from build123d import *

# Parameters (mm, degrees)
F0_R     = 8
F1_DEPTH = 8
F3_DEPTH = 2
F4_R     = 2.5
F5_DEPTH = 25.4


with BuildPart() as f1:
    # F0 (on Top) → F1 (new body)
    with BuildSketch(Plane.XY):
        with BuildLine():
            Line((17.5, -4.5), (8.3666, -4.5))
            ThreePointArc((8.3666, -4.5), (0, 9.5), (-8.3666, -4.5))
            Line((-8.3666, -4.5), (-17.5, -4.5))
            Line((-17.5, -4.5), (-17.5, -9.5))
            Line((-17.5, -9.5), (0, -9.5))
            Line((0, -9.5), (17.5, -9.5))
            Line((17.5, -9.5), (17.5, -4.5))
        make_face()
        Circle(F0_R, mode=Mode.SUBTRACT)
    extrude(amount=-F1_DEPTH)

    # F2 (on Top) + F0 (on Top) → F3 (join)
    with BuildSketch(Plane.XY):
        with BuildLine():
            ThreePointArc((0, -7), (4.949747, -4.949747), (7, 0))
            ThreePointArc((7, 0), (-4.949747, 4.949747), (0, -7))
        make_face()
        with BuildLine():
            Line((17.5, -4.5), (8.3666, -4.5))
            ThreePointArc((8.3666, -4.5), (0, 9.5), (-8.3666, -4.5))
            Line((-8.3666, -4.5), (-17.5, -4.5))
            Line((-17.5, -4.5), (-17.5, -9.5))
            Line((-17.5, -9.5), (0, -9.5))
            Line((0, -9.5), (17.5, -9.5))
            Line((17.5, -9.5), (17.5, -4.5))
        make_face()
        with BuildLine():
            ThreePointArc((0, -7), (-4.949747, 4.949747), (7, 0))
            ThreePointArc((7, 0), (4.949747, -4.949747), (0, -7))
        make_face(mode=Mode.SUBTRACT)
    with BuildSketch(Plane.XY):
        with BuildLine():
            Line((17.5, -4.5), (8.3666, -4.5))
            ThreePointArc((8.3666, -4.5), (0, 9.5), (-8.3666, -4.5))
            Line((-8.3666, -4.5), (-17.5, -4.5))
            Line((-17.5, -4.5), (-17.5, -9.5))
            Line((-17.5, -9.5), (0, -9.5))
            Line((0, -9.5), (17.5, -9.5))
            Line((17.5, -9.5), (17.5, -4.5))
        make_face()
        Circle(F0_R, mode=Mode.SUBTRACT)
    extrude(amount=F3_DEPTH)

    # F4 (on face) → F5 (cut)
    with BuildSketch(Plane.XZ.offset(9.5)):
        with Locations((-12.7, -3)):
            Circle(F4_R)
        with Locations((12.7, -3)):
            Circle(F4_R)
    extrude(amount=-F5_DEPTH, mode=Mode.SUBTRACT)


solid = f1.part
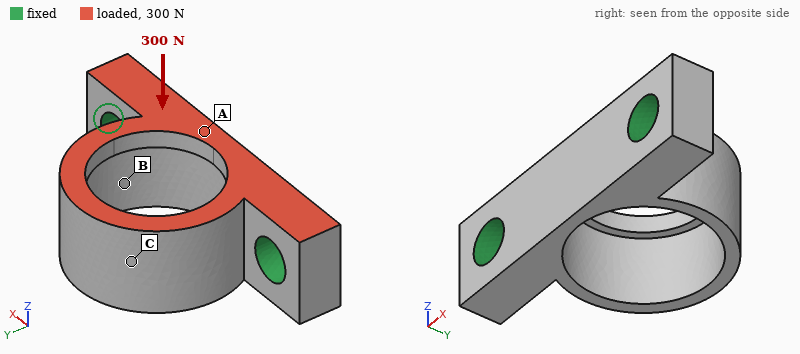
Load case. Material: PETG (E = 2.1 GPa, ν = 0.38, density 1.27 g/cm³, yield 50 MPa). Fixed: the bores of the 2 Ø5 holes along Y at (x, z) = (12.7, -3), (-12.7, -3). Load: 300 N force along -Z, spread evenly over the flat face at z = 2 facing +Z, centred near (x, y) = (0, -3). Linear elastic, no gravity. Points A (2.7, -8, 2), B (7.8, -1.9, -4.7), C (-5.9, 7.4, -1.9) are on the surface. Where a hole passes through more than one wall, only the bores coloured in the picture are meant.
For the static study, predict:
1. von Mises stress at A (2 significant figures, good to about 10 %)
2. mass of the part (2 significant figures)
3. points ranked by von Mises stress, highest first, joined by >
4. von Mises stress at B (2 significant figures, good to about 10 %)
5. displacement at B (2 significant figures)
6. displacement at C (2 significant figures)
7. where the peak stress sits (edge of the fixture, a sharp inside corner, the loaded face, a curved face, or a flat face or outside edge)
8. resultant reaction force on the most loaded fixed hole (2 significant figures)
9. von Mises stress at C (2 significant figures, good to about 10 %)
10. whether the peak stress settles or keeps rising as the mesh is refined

3.1 MPa
2.4 g
B > C > A
15 MPa
0.079 mm
0.30 mm
a sharp inside corner
150 N
8.5 MPa
keeps rising
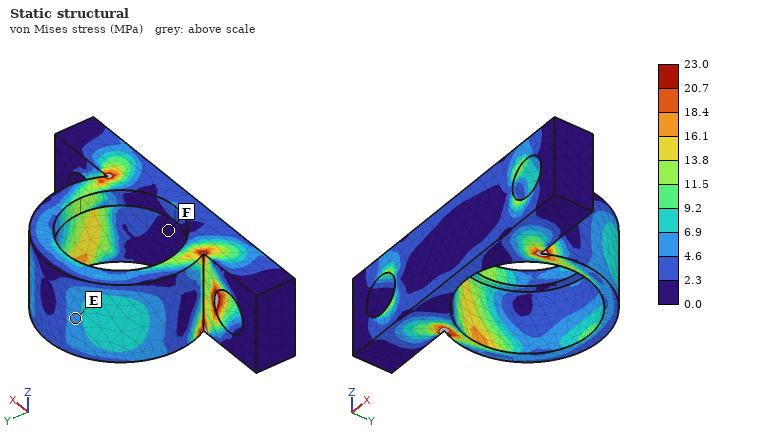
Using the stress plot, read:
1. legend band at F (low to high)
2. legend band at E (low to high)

0.0 to 2.3 MPa
4.6 to 6.9 MPa
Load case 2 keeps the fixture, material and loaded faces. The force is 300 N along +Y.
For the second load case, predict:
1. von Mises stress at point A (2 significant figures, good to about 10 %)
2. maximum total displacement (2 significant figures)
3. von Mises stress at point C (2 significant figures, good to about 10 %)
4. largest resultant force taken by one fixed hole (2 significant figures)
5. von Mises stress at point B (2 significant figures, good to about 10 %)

7.1 MPa
0.32 mm
4.7 MPa
150 N
7.2 MPa
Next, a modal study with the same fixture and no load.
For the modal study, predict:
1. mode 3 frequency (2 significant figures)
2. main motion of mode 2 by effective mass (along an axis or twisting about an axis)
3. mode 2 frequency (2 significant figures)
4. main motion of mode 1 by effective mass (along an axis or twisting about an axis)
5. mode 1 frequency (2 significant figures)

6100 Hz
along Z
3400 Hz
along X
2600 Hz
